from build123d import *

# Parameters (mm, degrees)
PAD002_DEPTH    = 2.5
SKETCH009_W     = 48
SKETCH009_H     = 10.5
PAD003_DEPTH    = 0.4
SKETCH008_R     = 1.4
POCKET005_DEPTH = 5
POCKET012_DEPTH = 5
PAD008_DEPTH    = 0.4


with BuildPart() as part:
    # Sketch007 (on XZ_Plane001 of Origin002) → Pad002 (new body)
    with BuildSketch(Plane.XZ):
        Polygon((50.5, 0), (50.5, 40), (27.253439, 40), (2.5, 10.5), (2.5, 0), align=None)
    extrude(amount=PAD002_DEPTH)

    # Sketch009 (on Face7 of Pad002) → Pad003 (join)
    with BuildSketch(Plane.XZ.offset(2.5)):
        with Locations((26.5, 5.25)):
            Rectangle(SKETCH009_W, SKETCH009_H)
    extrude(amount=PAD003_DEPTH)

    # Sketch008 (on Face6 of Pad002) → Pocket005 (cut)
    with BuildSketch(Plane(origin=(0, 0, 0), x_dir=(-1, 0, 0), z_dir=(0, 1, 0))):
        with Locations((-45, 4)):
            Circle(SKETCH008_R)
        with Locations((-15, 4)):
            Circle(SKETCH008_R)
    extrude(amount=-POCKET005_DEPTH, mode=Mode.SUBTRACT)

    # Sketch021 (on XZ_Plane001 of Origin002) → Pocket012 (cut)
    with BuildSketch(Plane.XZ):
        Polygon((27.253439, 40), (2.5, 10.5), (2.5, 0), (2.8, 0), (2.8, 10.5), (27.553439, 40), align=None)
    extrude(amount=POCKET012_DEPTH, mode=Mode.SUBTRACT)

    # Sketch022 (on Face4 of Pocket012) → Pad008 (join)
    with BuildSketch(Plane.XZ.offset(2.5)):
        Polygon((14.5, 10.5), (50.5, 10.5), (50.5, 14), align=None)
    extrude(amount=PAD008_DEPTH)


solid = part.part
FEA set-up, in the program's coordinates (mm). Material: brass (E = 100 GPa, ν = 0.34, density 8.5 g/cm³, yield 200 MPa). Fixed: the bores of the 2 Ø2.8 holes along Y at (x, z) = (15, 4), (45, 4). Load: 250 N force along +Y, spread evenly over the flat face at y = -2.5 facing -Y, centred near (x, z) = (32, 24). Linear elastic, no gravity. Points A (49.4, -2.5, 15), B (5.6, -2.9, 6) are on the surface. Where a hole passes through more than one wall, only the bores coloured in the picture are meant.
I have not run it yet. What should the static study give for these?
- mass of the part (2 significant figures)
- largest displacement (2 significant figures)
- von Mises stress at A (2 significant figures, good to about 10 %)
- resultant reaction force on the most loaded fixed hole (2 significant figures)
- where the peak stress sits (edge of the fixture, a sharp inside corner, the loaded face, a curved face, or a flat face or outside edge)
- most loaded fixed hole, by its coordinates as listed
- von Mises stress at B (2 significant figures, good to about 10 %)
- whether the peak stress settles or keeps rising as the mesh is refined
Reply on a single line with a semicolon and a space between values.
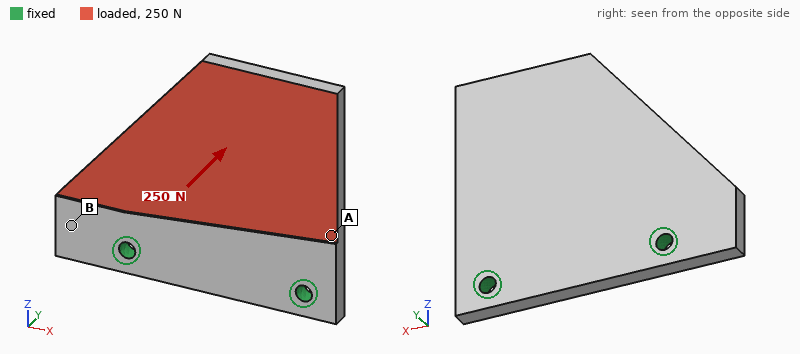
34 g; 0.30 mm; 78 MPa; 140 N; edge of the fixture; (45, 4); 22 MPa; keeps rising
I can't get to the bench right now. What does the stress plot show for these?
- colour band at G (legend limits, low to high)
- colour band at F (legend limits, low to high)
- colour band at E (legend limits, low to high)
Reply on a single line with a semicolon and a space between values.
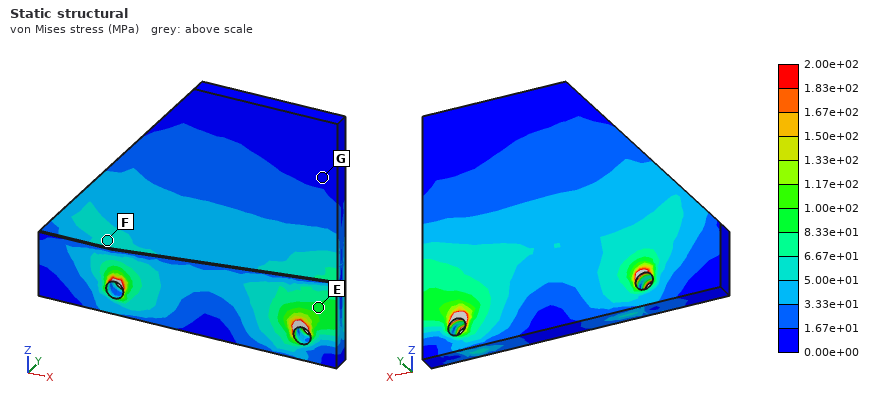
0.00e+00 to 1.67e+01 MPa; 5.00e+01 to 6.67e+01 MPa; 8.33e+01 to 1.00e+02 MPa
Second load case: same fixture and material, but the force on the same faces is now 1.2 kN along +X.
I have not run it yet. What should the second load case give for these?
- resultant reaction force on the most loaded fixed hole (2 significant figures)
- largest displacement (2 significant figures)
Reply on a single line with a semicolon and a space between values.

990 N; 55 µm
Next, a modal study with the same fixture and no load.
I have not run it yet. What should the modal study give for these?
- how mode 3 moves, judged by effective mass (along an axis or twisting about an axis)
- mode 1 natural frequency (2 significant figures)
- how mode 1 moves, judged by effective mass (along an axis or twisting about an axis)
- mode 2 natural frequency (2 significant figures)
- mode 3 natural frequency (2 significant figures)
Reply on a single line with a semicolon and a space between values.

along Y; 1300 Hz; along Y; 3600 Hz; 6600 Hz
